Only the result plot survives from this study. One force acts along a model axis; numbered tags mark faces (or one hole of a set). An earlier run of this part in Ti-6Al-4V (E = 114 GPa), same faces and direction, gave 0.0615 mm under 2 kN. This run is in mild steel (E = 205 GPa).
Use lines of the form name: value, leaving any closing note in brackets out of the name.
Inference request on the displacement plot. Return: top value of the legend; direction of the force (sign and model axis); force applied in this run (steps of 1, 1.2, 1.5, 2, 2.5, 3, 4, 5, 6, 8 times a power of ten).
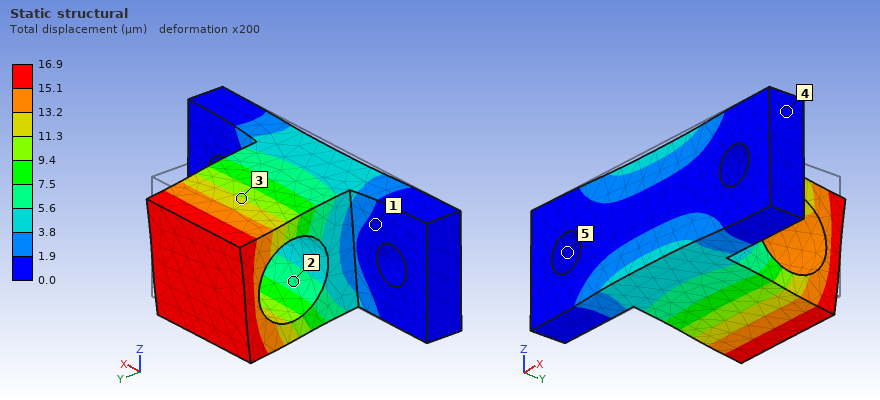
top value of the legend: 16.9 µm
direction of the force: -Z
force applied in this run: 1 kN
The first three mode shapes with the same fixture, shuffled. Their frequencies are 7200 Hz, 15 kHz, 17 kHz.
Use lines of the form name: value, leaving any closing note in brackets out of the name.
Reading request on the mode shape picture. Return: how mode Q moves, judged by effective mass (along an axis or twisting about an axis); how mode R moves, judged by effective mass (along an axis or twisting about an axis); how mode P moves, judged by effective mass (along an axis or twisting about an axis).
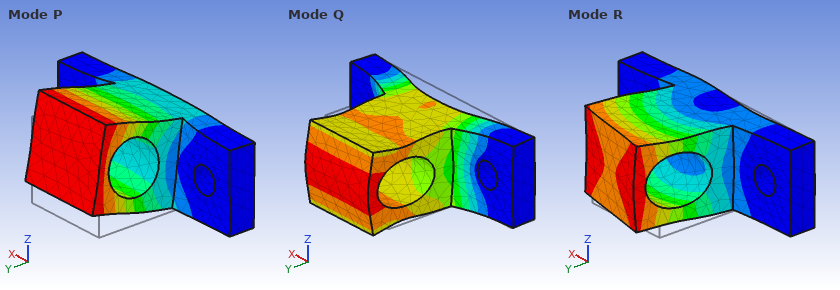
how mode Q moves, judged by effective mass: along Y
how mode R moves, judged by effective mass: along X
how mode P moves, judged by effective mass: along Z
